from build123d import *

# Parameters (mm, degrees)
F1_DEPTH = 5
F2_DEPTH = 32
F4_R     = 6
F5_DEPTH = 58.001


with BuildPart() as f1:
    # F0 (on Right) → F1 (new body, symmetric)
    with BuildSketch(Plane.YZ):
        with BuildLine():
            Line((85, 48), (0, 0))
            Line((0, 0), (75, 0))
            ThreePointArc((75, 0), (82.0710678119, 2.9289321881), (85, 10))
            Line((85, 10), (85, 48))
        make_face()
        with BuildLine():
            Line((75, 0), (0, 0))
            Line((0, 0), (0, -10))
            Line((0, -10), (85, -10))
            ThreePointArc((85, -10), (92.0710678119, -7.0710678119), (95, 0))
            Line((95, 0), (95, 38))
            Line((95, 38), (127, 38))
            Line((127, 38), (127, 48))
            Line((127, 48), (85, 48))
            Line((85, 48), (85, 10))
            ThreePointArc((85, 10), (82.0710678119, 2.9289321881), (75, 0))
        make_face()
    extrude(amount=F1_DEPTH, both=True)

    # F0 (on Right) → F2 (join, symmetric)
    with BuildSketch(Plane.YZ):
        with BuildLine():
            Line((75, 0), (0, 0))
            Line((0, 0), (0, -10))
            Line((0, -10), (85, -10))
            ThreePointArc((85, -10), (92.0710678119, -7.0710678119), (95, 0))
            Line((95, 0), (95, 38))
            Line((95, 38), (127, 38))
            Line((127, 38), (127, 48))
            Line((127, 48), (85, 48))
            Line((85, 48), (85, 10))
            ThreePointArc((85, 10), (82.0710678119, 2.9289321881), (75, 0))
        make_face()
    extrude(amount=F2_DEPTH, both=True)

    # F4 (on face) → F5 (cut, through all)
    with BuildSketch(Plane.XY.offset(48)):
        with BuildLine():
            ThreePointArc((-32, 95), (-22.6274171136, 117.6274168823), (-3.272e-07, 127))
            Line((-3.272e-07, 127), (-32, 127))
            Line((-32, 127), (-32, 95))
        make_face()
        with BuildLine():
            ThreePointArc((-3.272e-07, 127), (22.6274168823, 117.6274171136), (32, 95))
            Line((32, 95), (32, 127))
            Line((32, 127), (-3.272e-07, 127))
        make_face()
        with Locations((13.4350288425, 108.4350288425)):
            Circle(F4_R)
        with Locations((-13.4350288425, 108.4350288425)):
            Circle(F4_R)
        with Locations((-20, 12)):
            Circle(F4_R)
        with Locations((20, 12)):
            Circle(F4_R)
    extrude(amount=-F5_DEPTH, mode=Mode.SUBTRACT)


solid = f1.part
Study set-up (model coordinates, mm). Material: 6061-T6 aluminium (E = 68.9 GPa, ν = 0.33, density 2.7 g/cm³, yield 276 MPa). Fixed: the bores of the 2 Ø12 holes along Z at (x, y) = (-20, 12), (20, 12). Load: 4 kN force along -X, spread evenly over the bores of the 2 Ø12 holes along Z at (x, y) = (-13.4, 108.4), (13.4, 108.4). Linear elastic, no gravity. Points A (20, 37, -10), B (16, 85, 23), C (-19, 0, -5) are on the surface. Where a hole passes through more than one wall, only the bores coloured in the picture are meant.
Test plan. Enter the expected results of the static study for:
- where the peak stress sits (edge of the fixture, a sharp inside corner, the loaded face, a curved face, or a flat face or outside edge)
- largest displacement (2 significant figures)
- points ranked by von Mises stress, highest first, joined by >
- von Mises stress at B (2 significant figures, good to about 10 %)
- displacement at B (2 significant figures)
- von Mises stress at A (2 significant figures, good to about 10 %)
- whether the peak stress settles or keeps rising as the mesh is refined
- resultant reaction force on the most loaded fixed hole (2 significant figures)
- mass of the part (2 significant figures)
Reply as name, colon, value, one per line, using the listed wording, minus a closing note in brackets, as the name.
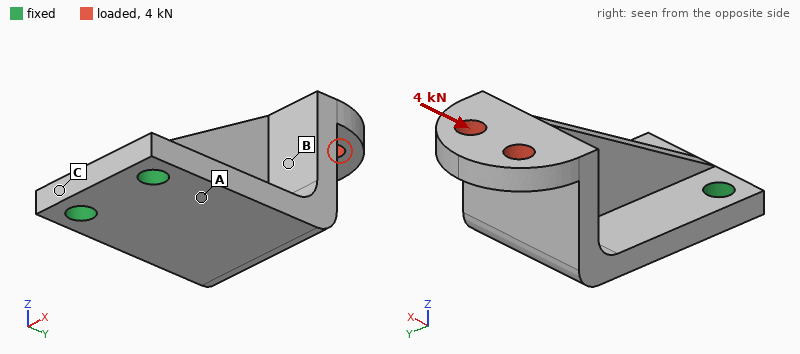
where the peak stress sits: edge of the fixture
largest displacement: 0.83 mm
points ranked by von Mises stress, highest first, joined by >: A > B > C
von Mises stress at B: 34 MPa
displacement at B: 0.43 mm
von Mises stress at A: 92 MPa
whether the peak stress settles or keeps rising as the mesh is refined: keeps rising
resultant reaction force on the most loaded fixed hole: 9.9 kN
mass of the part: 330 g
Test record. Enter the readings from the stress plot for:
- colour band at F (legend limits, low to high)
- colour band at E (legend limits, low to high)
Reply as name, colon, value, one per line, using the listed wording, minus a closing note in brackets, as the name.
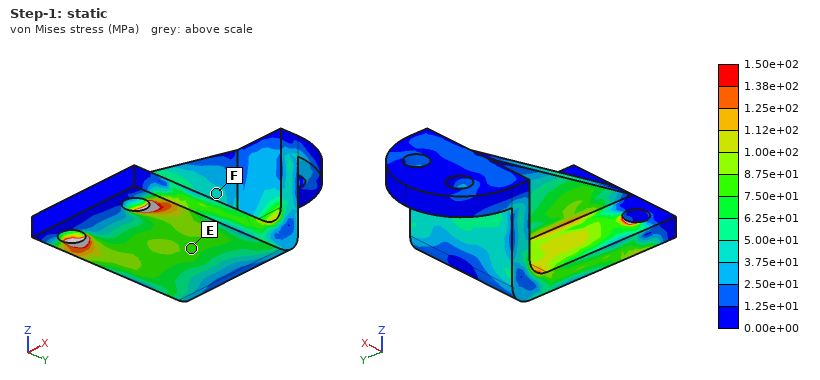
colour band at F: 3.75e+01 to 5.00e+01 MPa
colour band at E: 7.50e+01 to 8.75e+01 MPa
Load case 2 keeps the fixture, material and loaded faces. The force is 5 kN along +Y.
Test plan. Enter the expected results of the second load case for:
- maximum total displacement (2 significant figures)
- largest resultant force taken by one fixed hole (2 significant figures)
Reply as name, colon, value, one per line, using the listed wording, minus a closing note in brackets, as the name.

maximum total displacement: 1.0 mm
largest resultant force taken by one fixed hole: 2.5 kN
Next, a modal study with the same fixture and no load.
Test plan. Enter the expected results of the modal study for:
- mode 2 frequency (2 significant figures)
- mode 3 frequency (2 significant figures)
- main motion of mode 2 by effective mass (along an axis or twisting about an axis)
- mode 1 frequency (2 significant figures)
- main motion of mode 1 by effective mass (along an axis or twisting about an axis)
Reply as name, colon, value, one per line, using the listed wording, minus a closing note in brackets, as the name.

mode 2 frequency: 1200 Hz
mode 3 frequency: 3600 Hz
main motion of mode 2 by effective mass: along X
mode 1 frequency: 780 Hz
main motion of mode 1 by effective mass: along Z
